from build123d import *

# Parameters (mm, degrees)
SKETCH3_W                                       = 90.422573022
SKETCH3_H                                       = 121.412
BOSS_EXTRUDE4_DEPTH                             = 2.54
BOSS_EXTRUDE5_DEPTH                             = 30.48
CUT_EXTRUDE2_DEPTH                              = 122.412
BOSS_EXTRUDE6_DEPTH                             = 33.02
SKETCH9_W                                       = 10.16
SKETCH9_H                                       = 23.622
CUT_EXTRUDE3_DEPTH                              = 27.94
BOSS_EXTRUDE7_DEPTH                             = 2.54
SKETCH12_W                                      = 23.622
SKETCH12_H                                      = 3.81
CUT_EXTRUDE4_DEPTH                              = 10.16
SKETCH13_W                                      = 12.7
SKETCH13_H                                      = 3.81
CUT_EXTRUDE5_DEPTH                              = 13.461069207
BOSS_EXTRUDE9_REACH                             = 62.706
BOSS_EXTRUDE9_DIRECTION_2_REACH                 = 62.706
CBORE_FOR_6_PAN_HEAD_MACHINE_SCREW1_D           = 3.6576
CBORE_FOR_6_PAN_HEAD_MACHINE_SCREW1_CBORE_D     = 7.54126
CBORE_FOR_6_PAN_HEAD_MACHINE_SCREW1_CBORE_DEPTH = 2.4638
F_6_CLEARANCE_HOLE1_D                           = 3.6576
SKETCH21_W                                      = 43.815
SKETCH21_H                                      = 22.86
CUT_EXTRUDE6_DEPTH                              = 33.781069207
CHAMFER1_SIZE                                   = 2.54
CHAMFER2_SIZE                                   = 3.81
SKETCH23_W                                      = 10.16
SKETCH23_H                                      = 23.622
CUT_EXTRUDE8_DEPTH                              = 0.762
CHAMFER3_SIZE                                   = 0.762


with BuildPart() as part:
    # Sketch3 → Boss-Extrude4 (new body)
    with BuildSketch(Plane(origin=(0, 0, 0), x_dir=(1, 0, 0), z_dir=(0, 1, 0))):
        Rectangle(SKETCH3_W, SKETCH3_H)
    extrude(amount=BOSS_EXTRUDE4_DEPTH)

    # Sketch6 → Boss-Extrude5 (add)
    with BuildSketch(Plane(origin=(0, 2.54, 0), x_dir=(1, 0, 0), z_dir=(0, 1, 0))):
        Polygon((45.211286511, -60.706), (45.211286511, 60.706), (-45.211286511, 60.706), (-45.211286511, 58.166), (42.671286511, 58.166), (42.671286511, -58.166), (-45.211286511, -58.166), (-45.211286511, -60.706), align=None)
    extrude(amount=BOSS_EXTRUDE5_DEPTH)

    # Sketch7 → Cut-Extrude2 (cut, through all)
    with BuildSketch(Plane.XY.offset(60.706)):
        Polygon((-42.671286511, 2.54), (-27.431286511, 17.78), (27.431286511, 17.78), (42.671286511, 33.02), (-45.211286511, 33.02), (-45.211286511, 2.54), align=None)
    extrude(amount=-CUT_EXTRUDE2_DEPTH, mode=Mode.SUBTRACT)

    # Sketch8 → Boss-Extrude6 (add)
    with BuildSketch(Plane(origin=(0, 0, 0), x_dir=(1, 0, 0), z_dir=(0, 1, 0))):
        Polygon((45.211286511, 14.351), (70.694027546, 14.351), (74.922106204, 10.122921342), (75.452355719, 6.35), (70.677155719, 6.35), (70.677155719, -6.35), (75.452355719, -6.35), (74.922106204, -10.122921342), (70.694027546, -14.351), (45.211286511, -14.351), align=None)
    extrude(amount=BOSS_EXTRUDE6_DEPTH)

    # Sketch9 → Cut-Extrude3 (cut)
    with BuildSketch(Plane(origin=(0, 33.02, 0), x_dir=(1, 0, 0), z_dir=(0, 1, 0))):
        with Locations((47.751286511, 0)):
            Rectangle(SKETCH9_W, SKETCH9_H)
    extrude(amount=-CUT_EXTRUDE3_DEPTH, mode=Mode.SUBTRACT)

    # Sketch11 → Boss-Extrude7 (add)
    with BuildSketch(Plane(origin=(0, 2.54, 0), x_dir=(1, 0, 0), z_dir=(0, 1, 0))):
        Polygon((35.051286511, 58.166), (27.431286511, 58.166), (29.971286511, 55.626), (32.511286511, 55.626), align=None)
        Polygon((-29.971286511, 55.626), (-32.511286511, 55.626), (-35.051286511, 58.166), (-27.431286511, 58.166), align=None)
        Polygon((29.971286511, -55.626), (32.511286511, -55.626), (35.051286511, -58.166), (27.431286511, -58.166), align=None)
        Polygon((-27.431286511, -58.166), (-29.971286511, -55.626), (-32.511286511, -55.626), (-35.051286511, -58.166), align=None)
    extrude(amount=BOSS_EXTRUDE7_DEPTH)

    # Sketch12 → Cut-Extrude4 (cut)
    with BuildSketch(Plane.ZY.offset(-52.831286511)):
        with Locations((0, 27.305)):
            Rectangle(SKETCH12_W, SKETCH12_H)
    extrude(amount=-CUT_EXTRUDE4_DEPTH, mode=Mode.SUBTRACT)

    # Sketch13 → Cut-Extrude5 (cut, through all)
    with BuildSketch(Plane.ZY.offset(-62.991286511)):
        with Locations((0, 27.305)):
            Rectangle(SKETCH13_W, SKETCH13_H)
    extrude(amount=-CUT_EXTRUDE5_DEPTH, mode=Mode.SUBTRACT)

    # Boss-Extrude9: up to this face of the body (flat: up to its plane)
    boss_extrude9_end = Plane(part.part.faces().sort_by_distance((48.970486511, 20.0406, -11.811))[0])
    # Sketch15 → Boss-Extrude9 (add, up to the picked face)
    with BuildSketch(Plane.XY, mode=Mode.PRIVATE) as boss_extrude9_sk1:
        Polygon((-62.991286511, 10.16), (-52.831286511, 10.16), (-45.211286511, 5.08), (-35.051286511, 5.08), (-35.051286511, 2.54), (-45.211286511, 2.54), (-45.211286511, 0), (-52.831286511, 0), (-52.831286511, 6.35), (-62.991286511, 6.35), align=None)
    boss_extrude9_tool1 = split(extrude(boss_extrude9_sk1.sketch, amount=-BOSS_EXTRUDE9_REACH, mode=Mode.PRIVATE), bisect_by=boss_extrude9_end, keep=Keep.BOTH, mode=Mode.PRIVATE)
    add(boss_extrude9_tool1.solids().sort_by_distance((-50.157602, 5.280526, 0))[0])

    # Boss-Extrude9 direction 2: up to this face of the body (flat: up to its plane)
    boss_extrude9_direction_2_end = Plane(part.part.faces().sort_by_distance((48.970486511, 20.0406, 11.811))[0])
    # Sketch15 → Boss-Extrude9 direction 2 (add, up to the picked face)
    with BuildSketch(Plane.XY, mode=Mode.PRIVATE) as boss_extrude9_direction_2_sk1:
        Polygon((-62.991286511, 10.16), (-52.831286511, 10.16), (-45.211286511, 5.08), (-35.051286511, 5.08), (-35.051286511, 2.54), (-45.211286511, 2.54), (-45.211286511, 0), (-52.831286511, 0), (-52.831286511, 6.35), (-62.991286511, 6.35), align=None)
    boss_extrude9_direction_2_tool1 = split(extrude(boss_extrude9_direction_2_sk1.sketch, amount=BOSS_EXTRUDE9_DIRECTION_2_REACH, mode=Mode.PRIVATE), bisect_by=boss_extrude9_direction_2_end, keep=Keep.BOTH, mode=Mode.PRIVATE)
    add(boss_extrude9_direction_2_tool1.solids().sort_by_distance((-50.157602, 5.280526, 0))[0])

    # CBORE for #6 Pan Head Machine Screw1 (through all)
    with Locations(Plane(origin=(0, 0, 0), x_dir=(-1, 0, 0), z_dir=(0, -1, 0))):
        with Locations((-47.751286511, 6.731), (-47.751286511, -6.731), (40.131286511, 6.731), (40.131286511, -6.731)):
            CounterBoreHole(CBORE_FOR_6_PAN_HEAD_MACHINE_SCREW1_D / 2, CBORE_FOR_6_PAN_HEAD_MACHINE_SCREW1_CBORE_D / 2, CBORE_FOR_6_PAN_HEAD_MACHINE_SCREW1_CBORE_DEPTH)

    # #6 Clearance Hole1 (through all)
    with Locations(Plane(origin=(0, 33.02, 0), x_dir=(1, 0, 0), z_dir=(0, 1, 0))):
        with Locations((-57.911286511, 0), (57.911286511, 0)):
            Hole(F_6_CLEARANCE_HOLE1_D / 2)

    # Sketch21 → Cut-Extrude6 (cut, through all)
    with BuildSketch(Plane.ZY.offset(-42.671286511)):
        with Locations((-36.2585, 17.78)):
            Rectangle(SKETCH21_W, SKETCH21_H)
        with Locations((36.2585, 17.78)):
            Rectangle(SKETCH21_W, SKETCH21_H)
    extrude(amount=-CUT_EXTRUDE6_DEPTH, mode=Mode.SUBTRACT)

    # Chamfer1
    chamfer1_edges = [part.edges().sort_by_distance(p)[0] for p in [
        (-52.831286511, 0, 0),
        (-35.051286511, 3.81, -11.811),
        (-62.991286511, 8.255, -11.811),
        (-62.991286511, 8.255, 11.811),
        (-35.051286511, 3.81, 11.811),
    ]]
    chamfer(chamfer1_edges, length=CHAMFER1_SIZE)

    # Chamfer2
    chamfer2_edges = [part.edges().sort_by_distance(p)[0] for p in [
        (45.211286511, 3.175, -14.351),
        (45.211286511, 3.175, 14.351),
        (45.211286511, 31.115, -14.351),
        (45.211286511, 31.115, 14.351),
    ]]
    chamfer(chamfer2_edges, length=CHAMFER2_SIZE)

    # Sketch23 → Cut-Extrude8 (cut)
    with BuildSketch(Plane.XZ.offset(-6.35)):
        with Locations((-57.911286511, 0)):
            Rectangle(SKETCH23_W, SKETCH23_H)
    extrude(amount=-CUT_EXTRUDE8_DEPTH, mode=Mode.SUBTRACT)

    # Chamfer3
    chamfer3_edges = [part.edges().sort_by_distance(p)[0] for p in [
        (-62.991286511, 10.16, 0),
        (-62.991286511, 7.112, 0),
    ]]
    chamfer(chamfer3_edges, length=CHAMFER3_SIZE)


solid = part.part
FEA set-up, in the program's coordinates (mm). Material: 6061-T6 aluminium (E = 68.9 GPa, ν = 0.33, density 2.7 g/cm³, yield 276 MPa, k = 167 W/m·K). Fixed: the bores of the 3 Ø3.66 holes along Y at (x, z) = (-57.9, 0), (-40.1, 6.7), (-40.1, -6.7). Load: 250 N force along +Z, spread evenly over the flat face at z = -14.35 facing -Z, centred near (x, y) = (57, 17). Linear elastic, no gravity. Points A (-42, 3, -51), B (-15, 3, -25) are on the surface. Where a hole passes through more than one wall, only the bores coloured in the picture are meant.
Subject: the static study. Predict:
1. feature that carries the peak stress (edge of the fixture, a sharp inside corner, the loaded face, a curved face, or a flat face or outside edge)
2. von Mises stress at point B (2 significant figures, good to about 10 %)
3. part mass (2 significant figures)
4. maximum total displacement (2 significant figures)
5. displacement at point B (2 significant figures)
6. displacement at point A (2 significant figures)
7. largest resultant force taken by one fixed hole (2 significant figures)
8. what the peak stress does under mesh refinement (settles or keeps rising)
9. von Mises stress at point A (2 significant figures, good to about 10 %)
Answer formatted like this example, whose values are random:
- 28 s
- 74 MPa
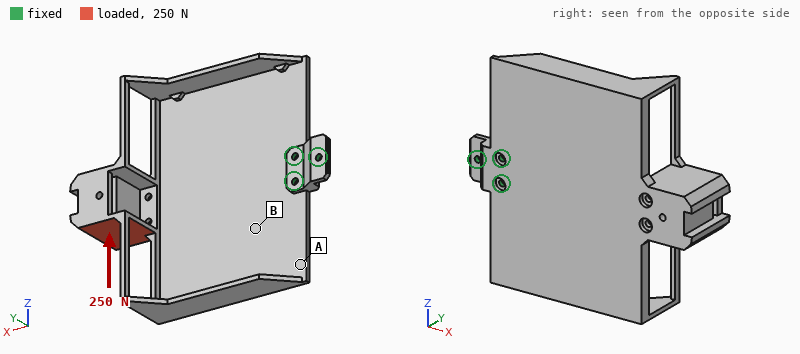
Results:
- edge of the fixture
- 22 MPa
- 160 g
- 1.3 mm
- 0.21 mm
- 0.33 mm
- 1.0 kN
- keeps rising
- 8.6 MPa
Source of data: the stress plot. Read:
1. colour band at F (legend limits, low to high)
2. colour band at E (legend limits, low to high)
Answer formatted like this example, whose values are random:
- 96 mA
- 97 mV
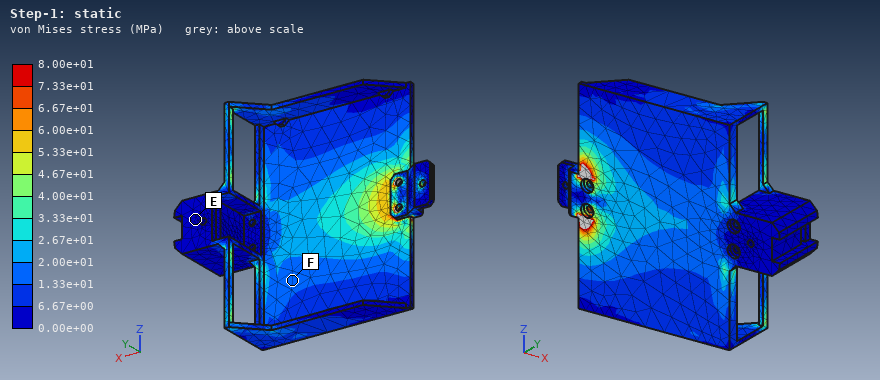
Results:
- 1.33e+01 to 2.00e+01 MPa
- 0.00e+00 to 6.67e+00 MPa
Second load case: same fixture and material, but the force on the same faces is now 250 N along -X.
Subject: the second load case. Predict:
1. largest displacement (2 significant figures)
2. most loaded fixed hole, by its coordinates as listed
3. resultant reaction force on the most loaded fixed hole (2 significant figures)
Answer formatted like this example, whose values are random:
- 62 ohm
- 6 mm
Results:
- 2.1 mm
- (-40.1, -6.7)
- 350 N
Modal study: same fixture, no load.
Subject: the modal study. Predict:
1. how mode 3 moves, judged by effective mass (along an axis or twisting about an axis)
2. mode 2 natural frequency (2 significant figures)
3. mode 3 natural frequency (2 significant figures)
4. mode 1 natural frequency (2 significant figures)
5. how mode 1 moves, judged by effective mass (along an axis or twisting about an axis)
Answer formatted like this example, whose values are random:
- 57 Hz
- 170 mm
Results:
- along Y
- 210 Hz
- 540 Hz
- 100 Hz
- along Y
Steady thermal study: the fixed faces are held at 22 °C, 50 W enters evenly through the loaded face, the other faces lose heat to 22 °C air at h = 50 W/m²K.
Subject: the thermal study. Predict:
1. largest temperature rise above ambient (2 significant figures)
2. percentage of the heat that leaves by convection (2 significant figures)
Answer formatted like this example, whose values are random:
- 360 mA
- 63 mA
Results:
- 66 K
- 84 %
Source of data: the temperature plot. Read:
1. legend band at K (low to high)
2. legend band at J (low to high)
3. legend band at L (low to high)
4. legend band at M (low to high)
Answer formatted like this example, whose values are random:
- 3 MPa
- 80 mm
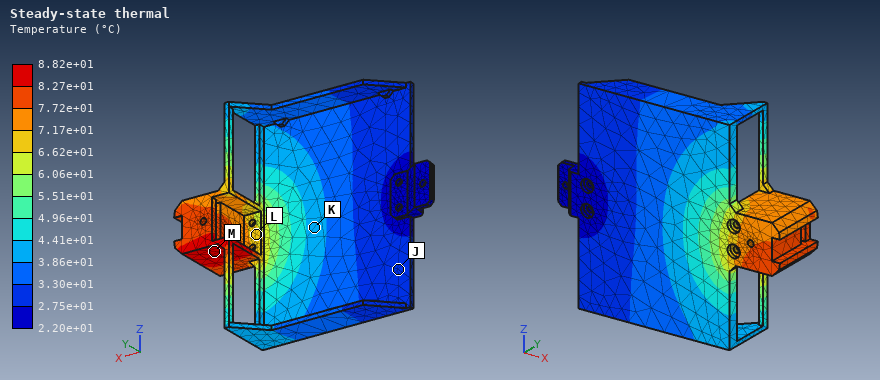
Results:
- 3.86e+01 to 4.41e+01 °C
- 2.75e+01 to 3.30e+01 °C
- 6.62e+01 to 7.17e+01 °C
- 8.27e+01 to 8.82e+01 °C
